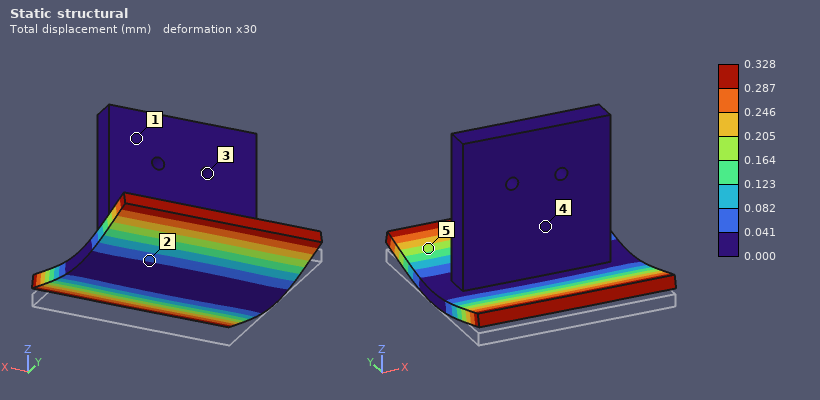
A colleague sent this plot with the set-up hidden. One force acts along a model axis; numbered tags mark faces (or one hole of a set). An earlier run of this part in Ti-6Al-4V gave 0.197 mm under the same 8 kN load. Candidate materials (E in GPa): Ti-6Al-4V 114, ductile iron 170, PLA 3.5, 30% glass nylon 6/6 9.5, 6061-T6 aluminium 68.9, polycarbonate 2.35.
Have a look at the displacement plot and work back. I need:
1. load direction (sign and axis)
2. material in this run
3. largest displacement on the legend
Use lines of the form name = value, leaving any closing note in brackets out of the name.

load direction = +Z
material in this run = 6061-T6 aluminium
largest displacement on the legend = 0.328 mm
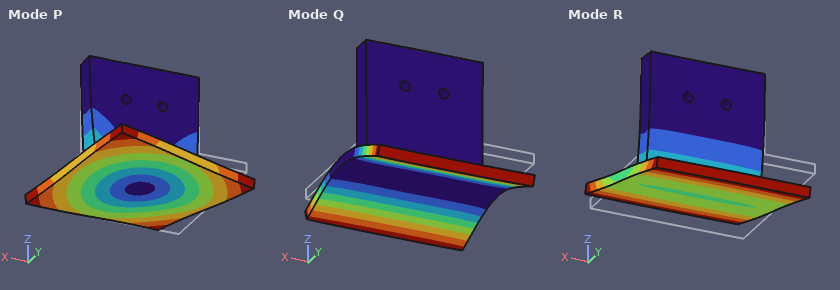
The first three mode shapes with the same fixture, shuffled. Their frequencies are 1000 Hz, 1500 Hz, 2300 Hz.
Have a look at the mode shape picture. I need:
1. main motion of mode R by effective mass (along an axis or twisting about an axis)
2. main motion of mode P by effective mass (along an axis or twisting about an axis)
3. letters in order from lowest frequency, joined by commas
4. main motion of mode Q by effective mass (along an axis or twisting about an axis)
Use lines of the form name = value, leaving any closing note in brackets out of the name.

main motion of mode R by effective mass = along Y
main motion of mode P by effective mass = twisting about Z
letters in order from lowest frequency, joined by commas = R, P, Q
main motion of mode Q by effective mass = along Z
